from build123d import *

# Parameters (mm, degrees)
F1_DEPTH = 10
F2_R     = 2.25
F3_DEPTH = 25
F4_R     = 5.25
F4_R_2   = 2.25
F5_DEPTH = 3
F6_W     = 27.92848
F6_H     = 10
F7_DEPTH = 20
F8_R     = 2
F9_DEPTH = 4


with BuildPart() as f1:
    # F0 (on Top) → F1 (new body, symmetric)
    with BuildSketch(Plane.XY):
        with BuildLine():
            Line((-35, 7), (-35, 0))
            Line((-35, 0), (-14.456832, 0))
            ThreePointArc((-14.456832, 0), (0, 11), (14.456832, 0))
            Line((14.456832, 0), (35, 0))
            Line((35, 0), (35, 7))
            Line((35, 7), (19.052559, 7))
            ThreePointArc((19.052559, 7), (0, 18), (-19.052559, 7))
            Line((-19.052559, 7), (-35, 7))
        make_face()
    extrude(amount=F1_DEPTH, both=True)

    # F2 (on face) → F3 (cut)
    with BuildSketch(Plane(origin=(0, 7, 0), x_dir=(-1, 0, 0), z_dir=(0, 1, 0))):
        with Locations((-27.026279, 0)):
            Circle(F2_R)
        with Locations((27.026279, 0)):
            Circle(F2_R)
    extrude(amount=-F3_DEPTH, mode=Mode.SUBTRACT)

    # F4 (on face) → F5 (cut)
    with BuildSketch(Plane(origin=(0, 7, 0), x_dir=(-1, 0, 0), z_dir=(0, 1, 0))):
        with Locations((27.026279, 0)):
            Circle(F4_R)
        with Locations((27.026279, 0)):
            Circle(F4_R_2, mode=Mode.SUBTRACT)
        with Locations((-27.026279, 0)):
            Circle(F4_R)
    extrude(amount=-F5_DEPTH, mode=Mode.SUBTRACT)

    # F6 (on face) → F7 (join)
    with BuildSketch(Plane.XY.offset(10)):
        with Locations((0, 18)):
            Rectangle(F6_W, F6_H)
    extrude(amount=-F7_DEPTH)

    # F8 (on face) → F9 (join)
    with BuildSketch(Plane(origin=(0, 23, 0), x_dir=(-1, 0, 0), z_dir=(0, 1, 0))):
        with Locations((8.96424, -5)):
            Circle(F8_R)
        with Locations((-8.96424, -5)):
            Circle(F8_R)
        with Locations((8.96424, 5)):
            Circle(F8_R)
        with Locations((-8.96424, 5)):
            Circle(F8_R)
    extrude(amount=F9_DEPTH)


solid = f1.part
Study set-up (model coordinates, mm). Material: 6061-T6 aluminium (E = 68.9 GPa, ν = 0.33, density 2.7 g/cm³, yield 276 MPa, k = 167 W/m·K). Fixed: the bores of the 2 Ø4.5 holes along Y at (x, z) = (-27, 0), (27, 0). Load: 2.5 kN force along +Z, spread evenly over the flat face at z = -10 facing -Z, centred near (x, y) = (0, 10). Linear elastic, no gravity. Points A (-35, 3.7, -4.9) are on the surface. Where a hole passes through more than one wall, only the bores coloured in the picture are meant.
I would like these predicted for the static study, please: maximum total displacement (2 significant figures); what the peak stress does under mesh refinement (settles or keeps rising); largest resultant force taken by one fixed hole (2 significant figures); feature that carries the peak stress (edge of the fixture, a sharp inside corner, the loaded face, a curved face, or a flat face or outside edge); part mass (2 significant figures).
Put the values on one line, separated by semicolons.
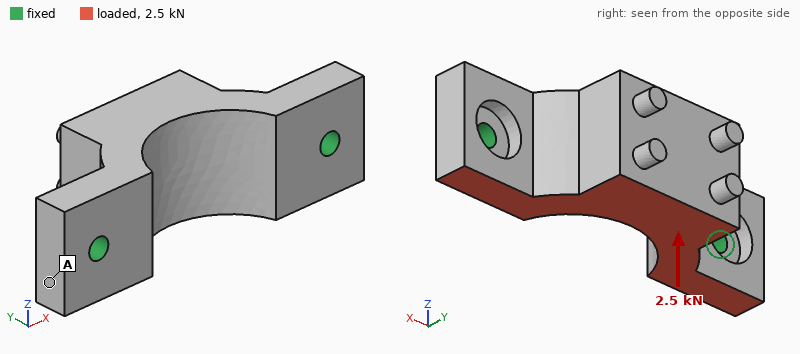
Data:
0.14 mm; keeps rising; 1.3 kN; edge of the fixture; 39 g
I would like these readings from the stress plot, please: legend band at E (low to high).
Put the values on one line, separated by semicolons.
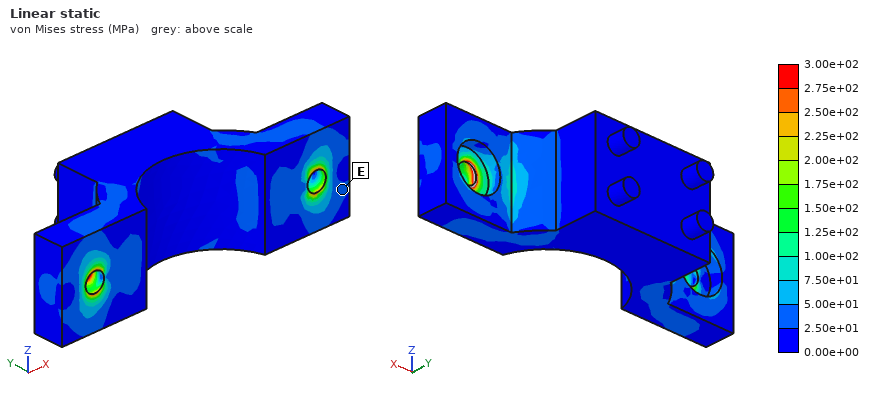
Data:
2.50e+01 to 5.00e+01 MPa
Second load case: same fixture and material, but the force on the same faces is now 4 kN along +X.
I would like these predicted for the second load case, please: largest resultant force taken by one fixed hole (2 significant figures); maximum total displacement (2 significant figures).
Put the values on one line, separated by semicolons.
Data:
2.2 kN; 17 µm
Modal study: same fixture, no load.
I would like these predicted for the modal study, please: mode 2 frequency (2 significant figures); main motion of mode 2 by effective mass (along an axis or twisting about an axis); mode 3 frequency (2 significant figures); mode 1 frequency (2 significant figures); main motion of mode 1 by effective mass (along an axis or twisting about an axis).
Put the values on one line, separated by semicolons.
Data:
11 kHz; along Y; 15 kHz; 4100 Hz; along Z
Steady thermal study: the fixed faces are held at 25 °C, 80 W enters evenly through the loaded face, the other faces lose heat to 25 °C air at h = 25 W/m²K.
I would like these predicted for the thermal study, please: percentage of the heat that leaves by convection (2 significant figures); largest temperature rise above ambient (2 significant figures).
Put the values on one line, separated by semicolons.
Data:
3.1 %; 36 K
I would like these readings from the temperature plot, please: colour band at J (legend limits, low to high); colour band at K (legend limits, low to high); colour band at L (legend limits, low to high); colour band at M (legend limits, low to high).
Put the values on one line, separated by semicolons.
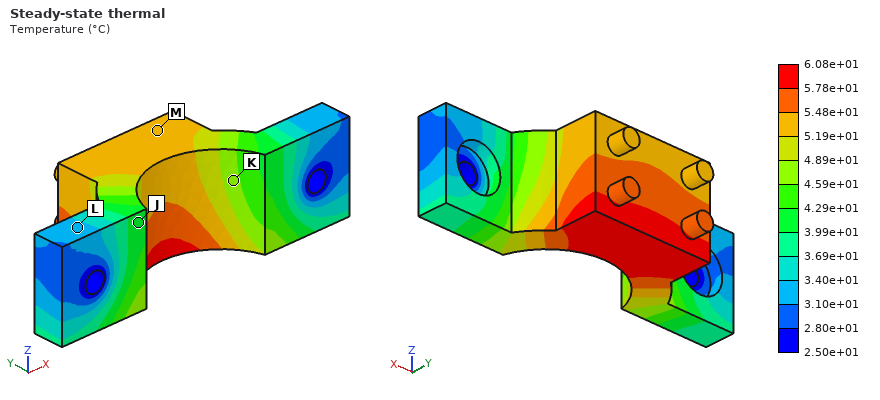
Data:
3.99e+01 to 4.29e+01 °C; 4.59e+01 to 4.89e+01 °C; 3.10e+01 to 3.40e+01 °C; 5.19e+01 to 5.48e+01 °C
